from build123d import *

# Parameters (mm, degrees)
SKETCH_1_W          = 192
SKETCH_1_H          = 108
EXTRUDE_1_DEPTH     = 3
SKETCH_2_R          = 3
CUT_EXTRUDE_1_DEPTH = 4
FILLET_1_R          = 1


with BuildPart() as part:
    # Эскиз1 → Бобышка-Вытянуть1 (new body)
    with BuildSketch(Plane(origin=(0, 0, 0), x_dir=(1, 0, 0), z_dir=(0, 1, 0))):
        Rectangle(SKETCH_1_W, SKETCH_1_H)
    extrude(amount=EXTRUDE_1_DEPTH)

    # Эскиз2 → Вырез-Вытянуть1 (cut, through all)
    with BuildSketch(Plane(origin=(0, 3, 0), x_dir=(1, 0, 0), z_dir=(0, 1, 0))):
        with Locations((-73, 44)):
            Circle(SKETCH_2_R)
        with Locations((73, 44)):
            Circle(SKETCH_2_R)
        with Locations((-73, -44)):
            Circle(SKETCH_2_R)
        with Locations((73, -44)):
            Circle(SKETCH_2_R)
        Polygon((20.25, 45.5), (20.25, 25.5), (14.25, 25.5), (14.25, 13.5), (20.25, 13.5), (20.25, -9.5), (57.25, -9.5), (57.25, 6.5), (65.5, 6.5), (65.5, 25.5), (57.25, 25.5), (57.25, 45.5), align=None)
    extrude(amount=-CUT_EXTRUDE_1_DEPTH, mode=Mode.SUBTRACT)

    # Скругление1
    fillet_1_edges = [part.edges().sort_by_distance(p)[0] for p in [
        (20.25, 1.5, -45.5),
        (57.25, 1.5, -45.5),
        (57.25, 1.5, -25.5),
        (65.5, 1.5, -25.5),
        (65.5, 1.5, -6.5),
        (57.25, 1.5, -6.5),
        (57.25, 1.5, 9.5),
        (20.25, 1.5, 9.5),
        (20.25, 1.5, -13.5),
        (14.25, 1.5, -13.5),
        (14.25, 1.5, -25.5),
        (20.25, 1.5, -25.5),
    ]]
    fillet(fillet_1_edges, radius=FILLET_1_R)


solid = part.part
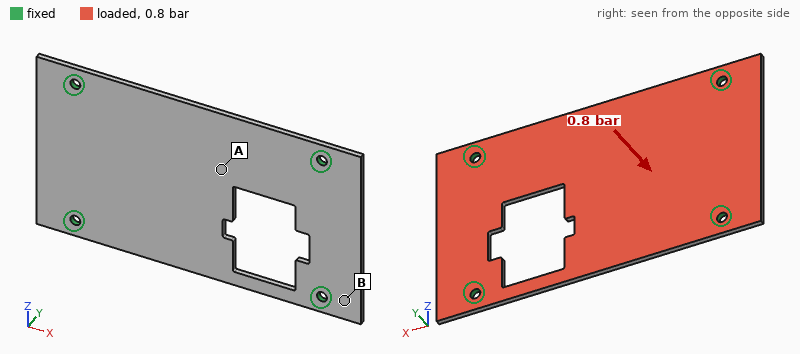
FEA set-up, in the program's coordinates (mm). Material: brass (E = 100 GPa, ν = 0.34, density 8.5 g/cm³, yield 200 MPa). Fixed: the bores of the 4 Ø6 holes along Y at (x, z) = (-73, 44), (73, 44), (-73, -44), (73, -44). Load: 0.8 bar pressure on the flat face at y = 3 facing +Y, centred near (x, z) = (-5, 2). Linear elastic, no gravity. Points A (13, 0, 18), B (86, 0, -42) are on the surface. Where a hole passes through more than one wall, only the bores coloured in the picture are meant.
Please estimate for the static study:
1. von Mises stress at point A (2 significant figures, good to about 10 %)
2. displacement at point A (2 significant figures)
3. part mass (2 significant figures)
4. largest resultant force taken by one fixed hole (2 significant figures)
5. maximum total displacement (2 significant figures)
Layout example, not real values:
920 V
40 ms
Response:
54 MPa
0.54 mm
470 g
400 N
0.65 mm
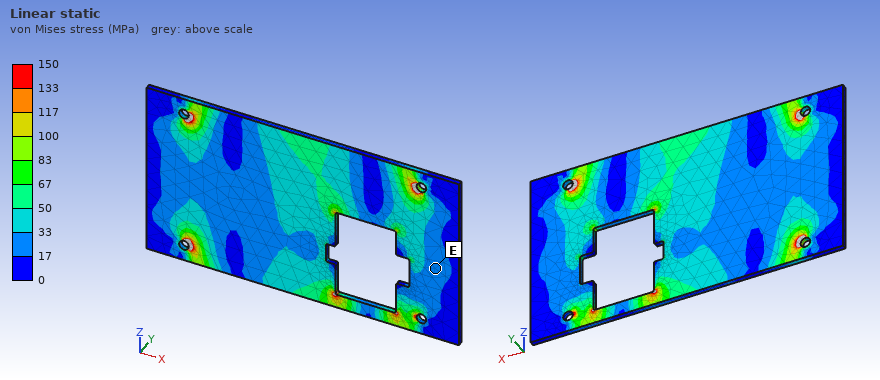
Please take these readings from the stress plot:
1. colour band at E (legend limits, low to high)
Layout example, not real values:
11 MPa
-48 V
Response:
17 to 33 MPa
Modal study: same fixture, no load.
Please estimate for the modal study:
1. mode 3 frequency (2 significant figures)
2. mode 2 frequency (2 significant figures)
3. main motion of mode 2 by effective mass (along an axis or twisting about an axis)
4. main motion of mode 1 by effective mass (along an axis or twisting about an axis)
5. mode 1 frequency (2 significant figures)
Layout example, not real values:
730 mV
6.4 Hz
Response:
1100 Hz
630 Hz
twisting about X
along Y
420 Hz
